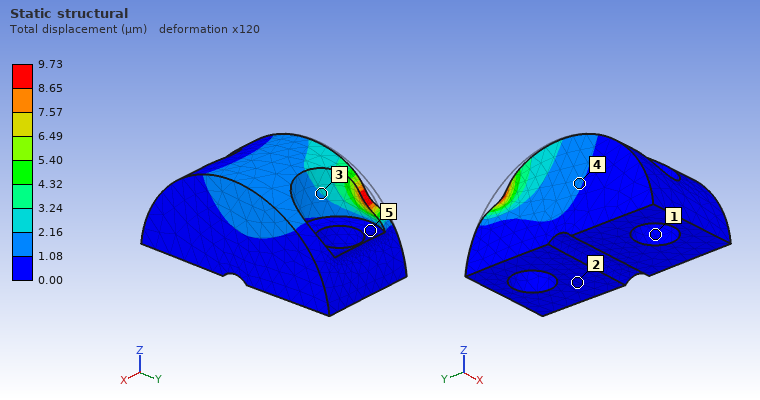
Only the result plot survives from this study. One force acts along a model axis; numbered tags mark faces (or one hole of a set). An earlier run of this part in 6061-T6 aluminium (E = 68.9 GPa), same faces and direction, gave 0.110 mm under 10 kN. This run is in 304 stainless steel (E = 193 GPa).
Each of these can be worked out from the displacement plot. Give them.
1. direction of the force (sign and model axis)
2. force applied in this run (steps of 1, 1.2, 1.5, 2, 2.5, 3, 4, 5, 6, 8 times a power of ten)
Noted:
+X
2.5 kN
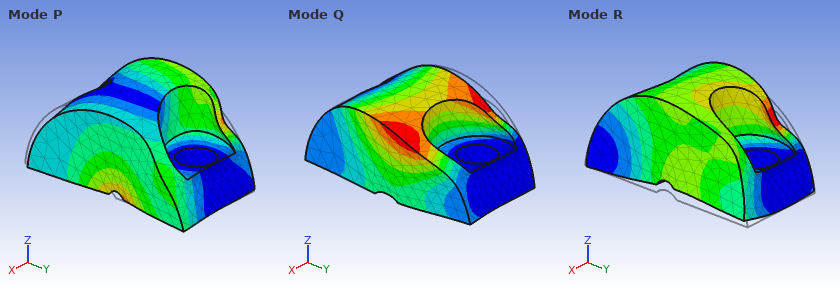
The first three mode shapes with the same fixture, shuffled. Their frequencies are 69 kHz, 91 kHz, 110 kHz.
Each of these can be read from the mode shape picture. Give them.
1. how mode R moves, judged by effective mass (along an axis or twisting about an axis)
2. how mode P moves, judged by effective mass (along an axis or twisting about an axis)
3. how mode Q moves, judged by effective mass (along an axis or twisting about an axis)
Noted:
along Z
along X
along X
